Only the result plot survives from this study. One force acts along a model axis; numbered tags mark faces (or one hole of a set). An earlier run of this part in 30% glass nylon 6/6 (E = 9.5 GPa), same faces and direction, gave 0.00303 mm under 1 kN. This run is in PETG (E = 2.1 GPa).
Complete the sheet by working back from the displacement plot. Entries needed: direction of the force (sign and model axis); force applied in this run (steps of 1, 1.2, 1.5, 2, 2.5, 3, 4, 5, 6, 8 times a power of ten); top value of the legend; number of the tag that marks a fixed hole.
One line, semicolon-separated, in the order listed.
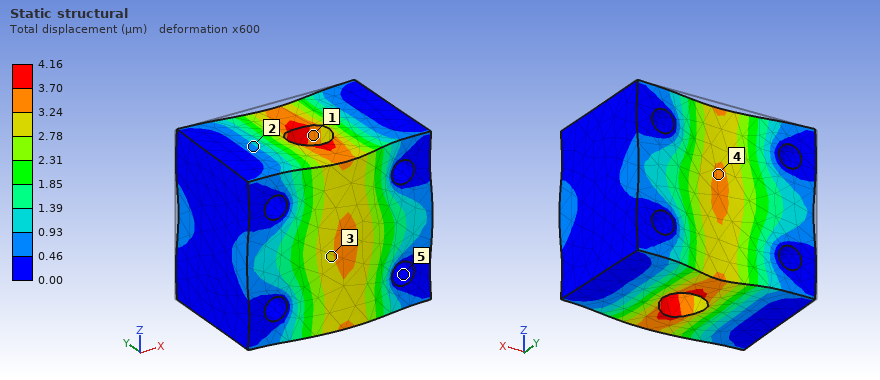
-Y; 300 N; 4.16 µm; 5
